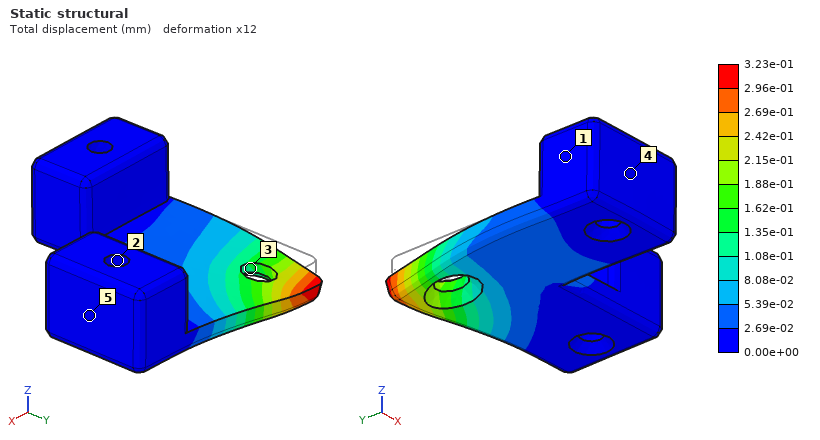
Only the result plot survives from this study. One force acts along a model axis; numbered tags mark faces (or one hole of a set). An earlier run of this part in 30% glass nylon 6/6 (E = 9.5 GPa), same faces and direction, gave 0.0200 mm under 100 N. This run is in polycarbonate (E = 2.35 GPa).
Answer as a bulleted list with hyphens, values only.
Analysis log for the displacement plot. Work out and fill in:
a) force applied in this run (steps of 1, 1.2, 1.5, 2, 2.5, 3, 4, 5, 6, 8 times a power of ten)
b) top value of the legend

- 400 N
- 3.23e-01 mm
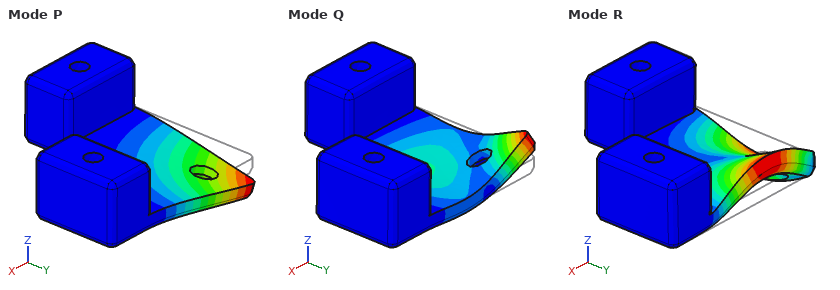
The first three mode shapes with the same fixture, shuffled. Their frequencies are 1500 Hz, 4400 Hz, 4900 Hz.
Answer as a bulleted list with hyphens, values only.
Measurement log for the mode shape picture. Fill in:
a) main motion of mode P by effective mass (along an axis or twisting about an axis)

- along Z
